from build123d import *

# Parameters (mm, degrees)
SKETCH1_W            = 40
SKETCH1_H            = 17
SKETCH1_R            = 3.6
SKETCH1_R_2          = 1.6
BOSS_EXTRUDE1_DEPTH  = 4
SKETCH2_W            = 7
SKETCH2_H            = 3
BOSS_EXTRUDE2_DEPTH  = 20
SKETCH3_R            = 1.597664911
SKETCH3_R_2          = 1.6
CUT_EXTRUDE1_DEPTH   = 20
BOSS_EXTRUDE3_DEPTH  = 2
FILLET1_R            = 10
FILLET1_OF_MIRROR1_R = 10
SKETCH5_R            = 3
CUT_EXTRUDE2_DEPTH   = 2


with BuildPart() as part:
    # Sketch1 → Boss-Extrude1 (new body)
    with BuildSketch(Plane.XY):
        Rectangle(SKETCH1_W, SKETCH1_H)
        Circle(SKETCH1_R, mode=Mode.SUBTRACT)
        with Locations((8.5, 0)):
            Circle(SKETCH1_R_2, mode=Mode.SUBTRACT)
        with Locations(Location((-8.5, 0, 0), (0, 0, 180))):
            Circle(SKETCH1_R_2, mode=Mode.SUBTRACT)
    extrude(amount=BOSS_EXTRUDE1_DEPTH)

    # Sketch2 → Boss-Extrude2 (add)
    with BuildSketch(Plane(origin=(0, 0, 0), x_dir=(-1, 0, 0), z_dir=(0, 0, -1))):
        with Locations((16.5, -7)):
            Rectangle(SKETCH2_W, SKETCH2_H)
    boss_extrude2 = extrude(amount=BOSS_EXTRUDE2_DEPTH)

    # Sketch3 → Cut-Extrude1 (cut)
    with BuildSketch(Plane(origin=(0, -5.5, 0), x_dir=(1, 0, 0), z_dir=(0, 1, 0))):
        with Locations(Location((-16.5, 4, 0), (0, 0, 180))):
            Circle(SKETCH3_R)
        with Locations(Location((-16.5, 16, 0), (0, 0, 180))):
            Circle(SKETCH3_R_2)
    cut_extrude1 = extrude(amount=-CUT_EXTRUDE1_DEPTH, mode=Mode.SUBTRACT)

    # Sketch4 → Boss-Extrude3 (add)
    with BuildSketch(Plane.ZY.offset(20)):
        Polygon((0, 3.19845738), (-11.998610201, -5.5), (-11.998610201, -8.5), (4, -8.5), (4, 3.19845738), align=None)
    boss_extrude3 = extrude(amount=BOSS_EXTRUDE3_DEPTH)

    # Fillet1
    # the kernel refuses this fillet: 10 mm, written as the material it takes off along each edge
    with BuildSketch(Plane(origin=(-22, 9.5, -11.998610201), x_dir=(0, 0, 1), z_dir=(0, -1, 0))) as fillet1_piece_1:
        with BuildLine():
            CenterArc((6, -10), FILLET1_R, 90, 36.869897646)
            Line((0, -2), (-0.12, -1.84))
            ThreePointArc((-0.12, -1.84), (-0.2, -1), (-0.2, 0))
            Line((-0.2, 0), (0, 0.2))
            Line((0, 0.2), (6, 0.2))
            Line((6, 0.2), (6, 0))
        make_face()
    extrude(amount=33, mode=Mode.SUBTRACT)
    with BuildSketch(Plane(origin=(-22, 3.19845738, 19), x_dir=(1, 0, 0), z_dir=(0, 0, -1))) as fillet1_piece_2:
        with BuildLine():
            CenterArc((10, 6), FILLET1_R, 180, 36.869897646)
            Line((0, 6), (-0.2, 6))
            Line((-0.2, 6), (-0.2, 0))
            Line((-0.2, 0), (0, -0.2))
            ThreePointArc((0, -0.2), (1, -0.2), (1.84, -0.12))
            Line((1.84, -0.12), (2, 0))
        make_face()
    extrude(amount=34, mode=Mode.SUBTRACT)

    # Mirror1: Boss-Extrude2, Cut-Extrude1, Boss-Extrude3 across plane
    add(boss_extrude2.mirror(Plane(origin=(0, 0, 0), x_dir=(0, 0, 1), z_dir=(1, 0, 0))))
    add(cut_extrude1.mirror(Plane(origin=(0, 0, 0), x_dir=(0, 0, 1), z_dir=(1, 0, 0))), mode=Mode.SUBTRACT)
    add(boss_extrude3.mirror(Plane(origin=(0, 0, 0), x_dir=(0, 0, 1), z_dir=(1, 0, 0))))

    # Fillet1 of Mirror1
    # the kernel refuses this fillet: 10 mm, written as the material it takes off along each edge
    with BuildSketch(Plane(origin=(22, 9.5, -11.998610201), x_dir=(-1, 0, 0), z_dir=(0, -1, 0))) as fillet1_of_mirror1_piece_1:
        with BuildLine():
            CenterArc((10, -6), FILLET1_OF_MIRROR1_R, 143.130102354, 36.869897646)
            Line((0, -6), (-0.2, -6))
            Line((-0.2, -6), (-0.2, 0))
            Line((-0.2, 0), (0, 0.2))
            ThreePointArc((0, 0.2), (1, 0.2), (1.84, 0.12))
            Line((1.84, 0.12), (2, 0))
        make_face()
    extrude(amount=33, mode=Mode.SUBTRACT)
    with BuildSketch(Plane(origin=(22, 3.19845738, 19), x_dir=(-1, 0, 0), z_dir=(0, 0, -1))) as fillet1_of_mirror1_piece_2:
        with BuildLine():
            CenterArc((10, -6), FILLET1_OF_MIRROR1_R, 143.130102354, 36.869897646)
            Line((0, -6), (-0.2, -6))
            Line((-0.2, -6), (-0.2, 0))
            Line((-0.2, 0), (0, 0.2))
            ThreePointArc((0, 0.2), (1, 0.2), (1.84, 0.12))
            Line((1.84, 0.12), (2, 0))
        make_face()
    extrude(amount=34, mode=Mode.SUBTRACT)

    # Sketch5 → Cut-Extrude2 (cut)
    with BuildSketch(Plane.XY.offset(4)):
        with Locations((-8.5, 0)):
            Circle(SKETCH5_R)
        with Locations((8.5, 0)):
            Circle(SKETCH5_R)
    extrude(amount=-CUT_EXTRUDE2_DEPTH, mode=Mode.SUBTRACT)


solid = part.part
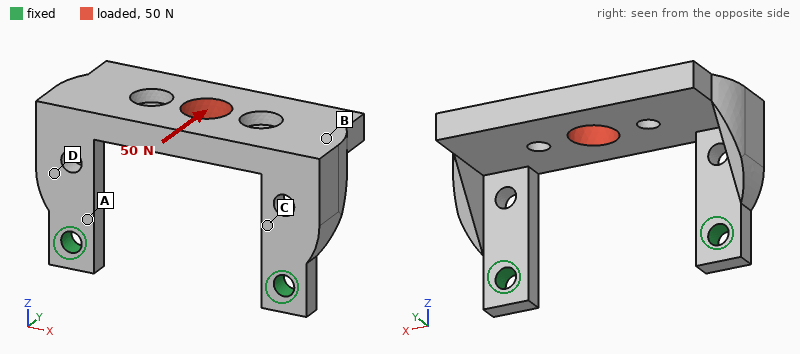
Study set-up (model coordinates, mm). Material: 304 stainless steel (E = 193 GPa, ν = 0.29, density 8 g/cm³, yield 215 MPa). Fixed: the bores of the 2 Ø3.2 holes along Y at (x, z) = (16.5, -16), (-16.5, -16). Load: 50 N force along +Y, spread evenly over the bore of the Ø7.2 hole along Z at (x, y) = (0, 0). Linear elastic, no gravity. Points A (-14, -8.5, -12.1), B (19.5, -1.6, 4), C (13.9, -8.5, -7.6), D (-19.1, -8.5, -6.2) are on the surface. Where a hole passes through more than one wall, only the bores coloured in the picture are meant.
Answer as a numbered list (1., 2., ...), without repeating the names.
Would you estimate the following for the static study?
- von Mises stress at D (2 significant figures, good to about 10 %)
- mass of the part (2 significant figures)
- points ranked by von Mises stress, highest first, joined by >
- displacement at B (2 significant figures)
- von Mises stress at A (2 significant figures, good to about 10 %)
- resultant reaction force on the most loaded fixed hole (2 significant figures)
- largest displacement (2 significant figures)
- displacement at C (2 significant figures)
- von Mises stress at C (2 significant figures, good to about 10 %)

1. 11 MPa
2. 29 g
3. A > C > D > B
4. 14 µm
5. 29 MPa
6. 25 N
7. 19 µm
8. 3.4 µm
9. 15 MPa
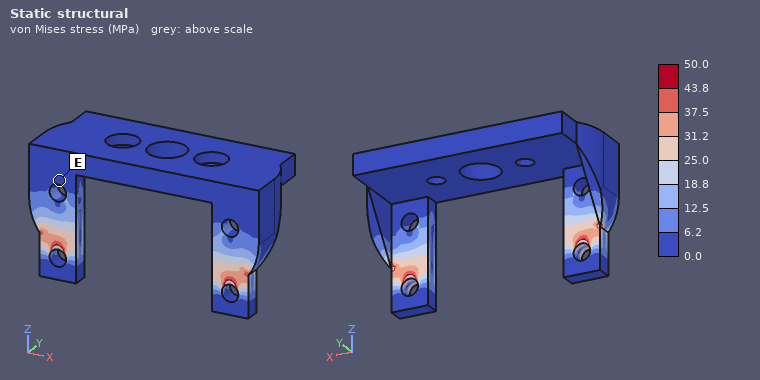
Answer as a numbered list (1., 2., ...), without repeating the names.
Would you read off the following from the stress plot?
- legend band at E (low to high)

1. 0.0 to 6.2 MPa
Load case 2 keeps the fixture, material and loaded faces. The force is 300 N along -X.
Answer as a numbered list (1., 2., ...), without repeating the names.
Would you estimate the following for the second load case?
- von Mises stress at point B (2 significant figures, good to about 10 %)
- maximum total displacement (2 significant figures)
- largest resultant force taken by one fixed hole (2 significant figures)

1. 18 MPa
2. 19 µm
3. 170 N
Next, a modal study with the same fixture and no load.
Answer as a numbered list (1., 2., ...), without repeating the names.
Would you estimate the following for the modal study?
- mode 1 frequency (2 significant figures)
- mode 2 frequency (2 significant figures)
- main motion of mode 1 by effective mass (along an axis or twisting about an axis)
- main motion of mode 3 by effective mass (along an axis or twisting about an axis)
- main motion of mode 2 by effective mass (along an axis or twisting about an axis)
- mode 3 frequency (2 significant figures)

1. 1900 Hz
2. 4100 Hz
3. along Y
4. along X
5. along X
6. 6000 Hz
